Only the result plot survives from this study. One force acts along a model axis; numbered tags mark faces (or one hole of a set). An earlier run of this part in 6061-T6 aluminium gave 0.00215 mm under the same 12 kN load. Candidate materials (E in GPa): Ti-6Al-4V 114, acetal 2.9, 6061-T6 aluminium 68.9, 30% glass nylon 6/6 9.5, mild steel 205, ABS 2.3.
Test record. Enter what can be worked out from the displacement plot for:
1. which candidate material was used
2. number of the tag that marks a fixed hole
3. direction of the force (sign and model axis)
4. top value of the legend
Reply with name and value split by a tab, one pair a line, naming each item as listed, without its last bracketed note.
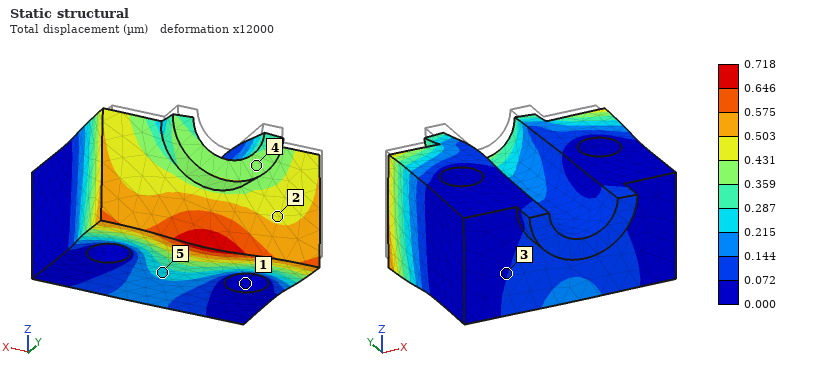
which candidate material was used	mild steel
number of the tag that marks a fixed hole	1
direction of the force	-Y
top value of the legend	0.718 µm
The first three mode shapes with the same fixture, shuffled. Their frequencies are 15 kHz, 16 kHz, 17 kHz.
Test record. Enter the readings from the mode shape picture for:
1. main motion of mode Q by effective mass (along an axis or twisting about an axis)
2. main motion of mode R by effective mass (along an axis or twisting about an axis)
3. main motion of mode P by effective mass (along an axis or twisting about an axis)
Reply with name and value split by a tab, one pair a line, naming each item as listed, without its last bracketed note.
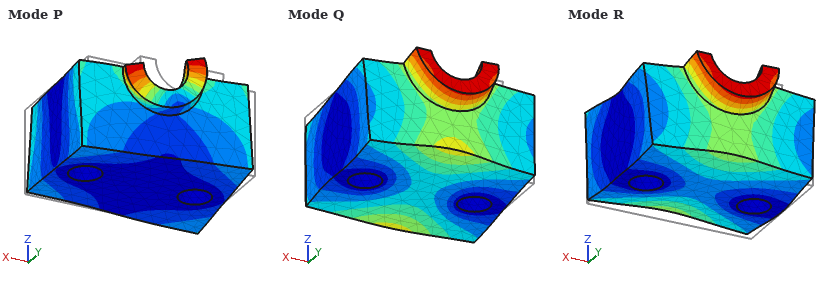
main motion of mode Q by effective mass	twisting about X
main motion of mode R by effective mass	along Z
main motion of mode P by effective mass	twisting about Z
